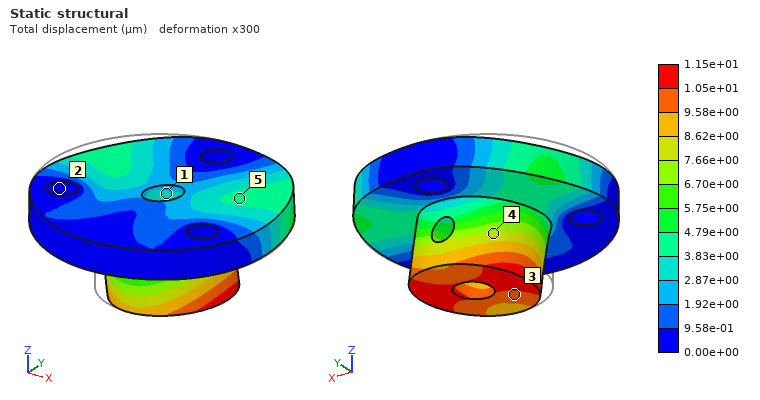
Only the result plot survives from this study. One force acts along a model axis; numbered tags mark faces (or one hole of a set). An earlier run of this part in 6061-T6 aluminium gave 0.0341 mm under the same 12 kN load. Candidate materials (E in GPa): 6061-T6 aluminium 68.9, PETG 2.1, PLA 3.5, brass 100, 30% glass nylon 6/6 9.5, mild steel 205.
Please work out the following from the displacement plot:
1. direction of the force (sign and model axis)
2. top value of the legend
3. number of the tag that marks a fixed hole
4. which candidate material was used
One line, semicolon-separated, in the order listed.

+X; 1.15e+01 µm; 2; mild steel
